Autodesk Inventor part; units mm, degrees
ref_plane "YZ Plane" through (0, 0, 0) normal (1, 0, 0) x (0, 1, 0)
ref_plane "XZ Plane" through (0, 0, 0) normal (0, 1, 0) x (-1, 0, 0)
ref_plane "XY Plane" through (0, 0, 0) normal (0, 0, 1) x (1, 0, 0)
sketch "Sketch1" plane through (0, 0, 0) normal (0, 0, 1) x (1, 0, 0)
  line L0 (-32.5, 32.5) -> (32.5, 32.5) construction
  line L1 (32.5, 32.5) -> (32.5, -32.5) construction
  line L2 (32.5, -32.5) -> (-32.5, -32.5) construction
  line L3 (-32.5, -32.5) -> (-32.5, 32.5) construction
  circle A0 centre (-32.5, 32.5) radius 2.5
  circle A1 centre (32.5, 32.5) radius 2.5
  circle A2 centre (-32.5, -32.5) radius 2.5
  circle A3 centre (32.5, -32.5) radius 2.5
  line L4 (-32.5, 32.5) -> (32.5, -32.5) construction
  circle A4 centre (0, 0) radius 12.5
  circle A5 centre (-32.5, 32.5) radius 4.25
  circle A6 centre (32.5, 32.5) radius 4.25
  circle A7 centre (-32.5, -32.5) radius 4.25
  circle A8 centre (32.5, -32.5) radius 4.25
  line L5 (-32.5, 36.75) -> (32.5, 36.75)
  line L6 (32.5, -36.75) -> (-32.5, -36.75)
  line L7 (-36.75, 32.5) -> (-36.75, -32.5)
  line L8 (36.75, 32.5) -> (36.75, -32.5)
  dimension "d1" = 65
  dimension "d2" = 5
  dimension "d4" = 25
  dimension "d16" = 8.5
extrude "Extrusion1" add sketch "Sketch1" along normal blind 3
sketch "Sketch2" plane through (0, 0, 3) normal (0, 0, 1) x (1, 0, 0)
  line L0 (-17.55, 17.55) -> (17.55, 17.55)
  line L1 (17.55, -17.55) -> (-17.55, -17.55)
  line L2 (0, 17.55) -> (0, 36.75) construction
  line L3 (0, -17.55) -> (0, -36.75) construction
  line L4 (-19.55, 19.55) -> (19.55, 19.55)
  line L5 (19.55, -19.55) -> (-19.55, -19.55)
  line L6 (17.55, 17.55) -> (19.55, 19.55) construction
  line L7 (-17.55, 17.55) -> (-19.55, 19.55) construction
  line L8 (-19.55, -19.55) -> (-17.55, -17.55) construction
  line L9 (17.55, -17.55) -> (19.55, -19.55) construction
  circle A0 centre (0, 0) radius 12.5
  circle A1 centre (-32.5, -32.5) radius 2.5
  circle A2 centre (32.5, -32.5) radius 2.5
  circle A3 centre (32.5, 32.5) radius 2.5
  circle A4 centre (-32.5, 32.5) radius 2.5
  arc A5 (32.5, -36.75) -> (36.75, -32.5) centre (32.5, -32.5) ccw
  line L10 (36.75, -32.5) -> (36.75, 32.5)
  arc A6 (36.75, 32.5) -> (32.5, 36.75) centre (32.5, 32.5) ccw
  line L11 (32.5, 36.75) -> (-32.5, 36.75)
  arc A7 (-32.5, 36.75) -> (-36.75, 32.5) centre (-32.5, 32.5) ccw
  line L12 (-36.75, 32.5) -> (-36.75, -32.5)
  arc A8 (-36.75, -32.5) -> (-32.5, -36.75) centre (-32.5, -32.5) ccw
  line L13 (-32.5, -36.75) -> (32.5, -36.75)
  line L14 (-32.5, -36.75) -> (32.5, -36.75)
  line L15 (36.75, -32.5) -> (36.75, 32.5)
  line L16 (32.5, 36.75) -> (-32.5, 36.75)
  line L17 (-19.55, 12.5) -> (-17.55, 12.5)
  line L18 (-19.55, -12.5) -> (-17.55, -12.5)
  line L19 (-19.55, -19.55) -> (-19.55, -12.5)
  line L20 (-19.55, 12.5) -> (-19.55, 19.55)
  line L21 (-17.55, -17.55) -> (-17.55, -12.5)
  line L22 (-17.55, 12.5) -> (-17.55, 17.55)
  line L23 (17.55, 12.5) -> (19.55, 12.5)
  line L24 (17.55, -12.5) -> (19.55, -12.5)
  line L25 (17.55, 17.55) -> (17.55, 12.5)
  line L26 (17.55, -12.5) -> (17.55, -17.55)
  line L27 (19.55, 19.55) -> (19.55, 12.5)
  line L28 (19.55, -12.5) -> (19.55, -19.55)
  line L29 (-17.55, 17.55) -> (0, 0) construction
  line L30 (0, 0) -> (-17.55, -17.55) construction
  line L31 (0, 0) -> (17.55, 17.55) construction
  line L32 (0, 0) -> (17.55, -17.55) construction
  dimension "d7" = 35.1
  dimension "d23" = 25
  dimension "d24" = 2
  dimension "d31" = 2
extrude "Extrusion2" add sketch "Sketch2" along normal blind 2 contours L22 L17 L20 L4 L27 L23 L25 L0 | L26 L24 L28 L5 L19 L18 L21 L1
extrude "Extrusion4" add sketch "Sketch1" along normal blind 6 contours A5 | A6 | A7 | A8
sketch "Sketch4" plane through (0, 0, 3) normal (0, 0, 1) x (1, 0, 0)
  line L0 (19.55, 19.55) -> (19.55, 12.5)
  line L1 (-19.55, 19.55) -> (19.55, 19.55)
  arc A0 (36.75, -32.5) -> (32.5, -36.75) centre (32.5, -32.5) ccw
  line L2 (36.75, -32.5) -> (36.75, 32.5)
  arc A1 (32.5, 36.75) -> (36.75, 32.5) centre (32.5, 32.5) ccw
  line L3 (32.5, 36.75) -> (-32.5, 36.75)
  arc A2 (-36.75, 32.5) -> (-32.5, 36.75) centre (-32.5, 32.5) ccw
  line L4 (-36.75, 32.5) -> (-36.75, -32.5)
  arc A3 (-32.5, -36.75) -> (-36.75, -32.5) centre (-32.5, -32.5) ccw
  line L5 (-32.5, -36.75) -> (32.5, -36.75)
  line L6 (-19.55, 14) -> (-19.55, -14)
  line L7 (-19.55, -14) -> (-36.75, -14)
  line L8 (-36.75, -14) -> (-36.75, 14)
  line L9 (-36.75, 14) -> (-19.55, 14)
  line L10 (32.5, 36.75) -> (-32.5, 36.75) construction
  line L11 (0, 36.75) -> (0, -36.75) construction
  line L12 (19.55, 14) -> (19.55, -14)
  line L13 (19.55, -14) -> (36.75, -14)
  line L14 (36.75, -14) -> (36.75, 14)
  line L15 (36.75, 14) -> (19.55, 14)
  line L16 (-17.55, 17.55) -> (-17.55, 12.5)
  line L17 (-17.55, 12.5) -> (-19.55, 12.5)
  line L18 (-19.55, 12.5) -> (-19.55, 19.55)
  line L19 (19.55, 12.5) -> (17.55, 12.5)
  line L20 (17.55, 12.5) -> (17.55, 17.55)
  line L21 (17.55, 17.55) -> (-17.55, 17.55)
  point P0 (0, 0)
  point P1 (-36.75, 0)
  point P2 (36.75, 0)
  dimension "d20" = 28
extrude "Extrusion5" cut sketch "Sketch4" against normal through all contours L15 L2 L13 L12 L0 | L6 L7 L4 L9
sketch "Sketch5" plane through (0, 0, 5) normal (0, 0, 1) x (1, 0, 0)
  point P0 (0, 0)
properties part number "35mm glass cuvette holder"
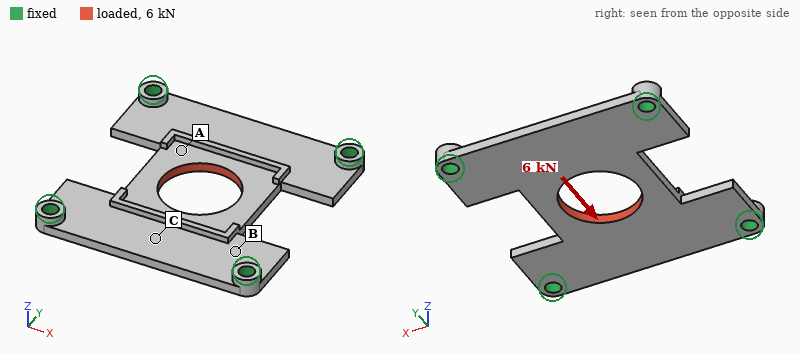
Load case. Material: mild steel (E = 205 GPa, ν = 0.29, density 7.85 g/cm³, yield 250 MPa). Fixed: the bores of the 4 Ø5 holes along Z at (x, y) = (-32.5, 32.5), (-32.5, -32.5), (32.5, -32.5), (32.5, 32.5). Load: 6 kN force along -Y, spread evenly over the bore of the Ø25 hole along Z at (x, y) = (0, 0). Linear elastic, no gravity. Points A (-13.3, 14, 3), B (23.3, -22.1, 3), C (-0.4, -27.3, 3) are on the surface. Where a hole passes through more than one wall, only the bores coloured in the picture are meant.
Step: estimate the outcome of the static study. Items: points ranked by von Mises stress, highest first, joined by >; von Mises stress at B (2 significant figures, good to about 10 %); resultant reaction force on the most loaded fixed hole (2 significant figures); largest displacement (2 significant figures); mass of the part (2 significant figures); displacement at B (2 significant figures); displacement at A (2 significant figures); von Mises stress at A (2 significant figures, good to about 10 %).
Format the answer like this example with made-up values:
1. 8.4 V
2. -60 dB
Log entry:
1. B > A > C
2. 53 MPa
3. 1.9 kN
4. 13 µm
5. 97 g
6. 5.4 µm
7. 10 µm
8. 31 MPa
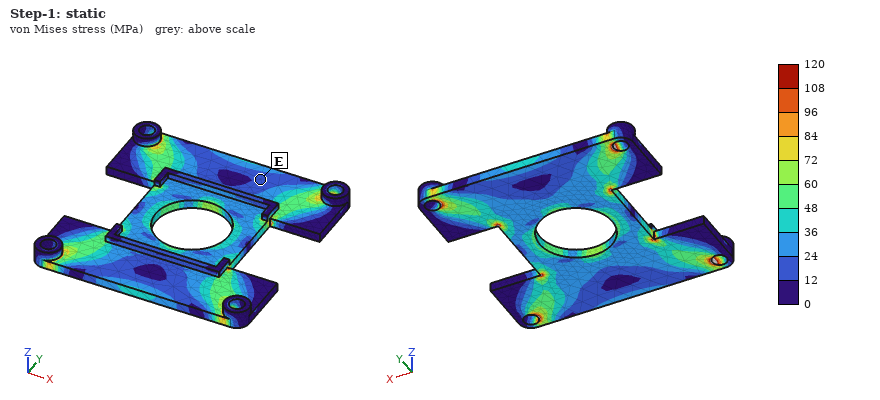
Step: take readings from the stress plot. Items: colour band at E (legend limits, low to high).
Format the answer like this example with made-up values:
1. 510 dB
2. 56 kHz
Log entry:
1. 12 to 24 MPa
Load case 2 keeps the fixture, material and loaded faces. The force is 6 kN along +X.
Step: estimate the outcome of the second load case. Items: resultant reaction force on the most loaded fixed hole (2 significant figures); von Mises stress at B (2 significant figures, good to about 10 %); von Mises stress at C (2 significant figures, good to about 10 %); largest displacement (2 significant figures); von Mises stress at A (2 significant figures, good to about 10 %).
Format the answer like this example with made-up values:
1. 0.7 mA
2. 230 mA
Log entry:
1. 1.7 kN
2. 38 MPa
3. 19 MPa
4. 13 µm
5. 37 MPa
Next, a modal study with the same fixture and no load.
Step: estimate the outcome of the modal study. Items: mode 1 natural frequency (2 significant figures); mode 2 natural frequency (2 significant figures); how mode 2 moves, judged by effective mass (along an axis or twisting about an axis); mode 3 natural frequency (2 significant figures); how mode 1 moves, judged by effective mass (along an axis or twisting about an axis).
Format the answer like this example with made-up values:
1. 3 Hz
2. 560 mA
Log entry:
1. 2800 Hz
2. 4300 Hz
3. twisting about X
4. 5600 Hz
5. along Z
